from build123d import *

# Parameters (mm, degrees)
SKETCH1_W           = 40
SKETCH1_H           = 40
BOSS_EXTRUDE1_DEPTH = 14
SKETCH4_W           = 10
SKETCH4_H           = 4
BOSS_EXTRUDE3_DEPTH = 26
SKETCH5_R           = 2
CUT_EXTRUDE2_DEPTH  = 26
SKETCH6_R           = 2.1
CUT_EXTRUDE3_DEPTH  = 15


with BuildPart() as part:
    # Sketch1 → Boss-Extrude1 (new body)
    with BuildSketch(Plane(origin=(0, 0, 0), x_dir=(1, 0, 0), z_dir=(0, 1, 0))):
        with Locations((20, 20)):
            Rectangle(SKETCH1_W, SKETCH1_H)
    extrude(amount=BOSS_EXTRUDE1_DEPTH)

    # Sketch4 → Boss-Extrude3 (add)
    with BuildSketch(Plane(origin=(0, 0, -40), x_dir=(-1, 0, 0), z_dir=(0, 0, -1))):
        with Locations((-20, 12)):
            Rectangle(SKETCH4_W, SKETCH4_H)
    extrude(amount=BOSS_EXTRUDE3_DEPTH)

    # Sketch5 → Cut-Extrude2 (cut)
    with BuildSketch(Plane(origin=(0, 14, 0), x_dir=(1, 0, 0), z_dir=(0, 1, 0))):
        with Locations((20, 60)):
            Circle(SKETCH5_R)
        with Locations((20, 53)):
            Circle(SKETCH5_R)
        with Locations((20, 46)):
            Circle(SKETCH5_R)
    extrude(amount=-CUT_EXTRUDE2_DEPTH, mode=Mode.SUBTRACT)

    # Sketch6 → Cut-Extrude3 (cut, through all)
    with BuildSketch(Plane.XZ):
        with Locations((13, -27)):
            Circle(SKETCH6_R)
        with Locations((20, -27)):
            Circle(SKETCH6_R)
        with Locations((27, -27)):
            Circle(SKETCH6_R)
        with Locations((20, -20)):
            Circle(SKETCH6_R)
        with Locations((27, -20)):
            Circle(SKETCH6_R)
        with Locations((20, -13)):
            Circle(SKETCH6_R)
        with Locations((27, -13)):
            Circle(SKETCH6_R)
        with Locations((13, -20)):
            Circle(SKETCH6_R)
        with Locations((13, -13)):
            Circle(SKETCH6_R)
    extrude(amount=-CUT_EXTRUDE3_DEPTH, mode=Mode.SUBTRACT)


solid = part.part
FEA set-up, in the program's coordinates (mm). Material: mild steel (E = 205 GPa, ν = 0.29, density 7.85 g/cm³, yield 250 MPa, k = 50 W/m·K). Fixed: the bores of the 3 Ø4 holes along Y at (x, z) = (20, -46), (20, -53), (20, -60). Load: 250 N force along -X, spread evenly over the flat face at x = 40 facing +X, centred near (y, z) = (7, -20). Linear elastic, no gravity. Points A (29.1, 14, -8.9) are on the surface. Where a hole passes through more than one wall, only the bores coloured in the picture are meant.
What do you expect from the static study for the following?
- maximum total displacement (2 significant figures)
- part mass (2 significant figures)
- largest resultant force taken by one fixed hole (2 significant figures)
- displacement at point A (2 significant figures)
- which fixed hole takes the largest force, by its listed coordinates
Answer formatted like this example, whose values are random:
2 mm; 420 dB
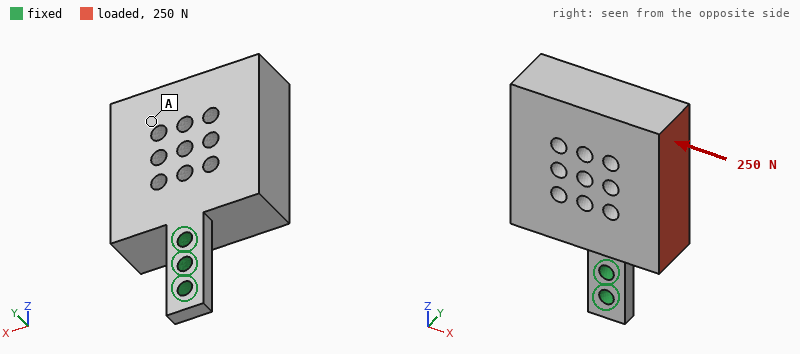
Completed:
45 µm; 170 g; 510 N; 30 µm; (20, -46)
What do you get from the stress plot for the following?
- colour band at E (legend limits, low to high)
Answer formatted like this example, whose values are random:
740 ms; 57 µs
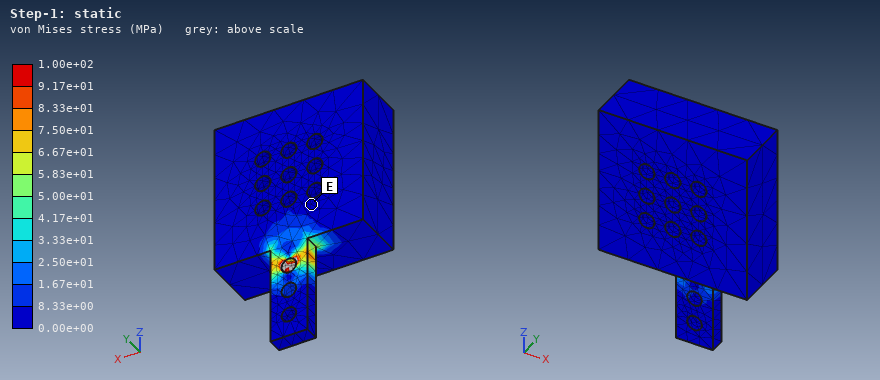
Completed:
0.00e+00 to 8.33e+00 MPa
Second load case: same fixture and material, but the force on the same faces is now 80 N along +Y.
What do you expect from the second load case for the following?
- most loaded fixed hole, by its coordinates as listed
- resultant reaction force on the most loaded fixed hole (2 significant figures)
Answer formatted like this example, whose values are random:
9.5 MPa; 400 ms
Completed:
(20, -46); 110 N
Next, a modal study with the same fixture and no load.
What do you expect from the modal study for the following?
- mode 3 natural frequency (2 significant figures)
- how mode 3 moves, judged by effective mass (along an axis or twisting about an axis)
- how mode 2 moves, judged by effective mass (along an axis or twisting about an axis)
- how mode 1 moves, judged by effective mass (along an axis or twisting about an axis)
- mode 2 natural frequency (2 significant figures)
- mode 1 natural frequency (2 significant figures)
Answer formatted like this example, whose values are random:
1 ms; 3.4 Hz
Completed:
1600 Hz; twisting about Z; along X; along Y; 1100 Hz; 630 Hz
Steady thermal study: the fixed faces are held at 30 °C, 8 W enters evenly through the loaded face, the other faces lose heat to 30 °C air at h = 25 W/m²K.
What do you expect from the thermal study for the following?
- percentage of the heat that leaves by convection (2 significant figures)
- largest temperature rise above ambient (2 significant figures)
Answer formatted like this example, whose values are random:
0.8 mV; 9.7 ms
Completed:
41 %; 27 K
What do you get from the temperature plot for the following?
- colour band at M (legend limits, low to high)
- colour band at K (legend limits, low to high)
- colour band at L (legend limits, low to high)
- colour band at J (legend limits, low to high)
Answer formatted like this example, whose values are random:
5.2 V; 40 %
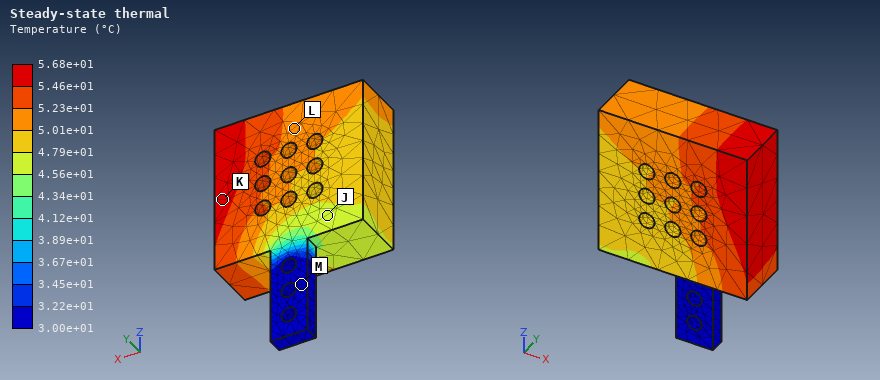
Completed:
3.00e+01 to 3.22e+01 °C; 5.46e+01 to 5.68e+01 °C; 5.01e+01 to 5.23e+01 °C; 4.56e+01 to 4.79e+01 °C
